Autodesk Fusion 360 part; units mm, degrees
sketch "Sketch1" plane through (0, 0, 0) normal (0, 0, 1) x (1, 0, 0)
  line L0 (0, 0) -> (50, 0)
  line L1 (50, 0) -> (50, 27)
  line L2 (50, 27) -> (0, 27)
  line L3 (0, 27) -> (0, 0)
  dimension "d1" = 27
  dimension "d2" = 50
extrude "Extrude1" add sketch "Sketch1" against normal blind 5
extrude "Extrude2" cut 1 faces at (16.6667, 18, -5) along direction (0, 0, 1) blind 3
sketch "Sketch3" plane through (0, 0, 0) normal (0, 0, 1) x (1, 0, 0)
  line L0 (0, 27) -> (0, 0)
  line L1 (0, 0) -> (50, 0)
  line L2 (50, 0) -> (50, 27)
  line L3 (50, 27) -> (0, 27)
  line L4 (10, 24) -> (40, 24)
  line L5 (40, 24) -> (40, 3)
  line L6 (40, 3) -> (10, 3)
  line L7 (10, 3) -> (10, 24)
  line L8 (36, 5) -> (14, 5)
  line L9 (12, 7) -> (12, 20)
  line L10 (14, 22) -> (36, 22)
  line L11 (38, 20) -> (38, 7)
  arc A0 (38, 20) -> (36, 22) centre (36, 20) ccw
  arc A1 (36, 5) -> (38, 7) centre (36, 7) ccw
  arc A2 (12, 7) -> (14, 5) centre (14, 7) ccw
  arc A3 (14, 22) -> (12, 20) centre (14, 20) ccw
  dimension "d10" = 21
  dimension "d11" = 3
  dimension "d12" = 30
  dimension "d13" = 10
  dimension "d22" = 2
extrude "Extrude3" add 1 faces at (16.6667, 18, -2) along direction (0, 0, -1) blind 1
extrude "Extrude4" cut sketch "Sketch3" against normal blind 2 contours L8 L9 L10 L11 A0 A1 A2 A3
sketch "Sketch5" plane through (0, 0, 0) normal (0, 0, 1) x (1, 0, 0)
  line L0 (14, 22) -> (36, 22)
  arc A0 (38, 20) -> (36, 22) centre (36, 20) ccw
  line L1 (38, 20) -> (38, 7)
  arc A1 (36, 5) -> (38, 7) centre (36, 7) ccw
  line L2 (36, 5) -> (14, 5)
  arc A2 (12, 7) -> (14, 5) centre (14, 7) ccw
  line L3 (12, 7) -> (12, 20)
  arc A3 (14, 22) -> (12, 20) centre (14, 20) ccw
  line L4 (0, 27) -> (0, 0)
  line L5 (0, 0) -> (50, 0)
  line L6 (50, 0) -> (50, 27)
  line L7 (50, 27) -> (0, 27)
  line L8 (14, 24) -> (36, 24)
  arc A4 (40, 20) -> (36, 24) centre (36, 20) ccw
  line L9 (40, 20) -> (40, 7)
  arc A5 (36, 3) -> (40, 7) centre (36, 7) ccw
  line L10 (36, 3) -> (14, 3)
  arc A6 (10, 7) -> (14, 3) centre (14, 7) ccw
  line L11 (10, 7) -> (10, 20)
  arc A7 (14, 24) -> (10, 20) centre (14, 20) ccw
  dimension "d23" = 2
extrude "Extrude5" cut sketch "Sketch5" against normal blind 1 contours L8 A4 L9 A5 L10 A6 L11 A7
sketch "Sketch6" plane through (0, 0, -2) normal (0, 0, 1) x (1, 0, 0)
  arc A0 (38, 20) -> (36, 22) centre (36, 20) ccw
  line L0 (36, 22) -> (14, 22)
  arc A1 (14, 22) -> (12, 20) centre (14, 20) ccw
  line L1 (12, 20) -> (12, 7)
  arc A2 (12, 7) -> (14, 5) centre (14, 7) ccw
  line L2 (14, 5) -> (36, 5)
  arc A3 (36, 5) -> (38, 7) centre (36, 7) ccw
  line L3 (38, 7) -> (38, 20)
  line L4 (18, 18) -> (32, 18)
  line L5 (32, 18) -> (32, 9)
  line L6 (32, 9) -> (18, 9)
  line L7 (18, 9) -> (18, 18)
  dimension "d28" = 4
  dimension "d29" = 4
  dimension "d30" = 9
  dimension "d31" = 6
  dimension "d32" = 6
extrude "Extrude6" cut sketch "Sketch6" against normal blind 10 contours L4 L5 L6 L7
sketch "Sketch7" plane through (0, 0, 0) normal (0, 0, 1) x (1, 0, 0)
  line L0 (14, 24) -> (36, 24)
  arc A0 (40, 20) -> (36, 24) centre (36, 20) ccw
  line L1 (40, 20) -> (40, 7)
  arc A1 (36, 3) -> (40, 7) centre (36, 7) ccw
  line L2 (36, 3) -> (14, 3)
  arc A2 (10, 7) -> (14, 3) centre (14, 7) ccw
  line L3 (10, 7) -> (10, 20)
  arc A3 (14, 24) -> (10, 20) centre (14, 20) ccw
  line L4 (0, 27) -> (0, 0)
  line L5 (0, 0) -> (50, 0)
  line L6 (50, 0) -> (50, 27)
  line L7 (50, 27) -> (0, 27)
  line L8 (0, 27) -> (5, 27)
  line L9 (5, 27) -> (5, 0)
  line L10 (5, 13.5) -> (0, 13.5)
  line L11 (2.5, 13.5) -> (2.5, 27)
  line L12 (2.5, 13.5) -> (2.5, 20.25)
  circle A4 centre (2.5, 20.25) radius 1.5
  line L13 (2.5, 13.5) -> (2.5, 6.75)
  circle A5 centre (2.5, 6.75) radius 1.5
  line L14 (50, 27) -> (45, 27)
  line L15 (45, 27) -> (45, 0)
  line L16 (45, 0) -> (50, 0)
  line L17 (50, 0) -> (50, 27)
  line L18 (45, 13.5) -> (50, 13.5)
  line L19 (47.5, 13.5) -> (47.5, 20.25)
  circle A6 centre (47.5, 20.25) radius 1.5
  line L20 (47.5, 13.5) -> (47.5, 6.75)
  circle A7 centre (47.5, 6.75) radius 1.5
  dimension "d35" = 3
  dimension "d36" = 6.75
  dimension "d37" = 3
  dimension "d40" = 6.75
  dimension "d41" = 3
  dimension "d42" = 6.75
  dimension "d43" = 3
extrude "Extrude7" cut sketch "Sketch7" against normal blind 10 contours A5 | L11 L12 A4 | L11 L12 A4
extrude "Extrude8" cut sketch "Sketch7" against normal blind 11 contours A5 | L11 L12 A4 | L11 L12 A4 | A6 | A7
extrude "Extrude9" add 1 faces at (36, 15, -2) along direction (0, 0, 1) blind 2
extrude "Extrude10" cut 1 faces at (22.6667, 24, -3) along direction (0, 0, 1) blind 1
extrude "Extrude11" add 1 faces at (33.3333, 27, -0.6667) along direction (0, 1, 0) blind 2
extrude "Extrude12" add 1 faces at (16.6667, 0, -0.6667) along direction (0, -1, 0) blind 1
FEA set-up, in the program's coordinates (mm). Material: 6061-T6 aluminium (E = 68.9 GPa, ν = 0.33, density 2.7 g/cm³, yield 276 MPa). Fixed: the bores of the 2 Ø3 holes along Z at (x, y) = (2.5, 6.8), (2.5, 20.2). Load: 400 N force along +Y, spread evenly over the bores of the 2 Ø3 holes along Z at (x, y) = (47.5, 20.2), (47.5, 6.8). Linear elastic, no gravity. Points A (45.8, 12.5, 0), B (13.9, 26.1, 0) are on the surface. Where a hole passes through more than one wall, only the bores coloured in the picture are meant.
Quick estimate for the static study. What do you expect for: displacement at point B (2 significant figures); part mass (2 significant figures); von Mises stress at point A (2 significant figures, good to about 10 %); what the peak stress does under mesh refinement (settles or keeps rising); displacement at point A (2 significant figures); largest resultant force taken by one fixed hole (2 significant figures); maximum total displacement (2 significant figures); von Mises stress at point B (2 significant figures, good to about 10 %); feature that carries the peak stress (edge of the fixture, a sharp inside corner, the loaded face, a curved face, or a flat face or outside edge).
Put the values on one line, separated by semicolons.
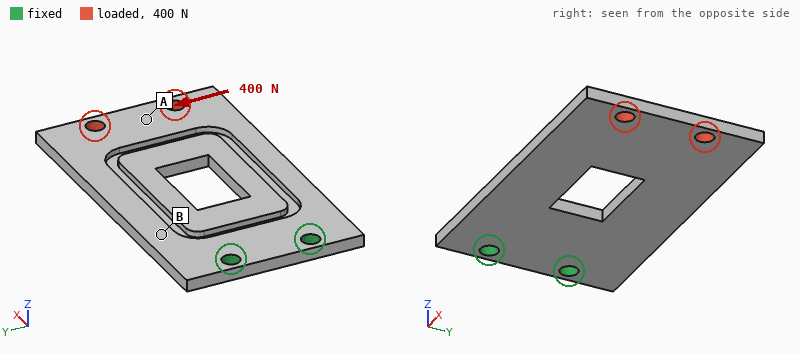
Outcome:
0.029 mm; 6.8 g; 18 MPa; keeps rising; 0.12 mm; 1.1 kN; 0.14 mm; 44 MPa; edge of the fixture
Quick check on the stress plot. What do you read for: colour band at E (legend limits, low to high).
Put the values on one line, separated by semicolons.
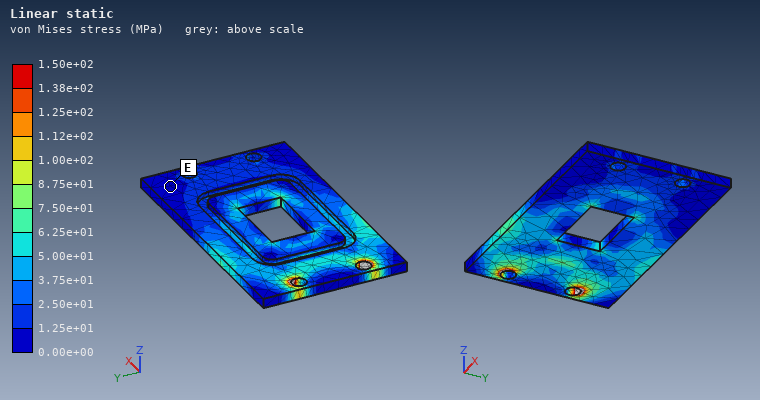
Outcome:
0.00e+00 to 1.25e+01 MPa
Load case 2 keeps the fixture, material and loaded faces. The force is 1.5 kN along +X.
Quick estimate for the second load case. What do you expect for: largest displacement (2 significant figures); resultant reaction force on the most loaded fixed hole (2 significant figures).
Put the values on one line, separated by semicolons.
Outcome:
0.21 mm; 760 N
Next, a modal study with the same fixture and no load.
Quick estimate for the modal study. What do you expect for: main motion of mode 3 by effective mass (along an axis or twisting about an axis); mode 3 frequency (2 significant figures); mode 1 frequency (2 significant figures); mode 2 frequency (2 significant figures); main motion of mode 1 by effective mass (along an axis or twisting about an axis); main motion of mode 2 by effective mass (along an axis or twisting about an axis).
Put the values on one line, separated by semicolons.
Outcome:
along Z; 4300 Hz; 650 Hz; 2100 Hz; along Z; twisting about X
